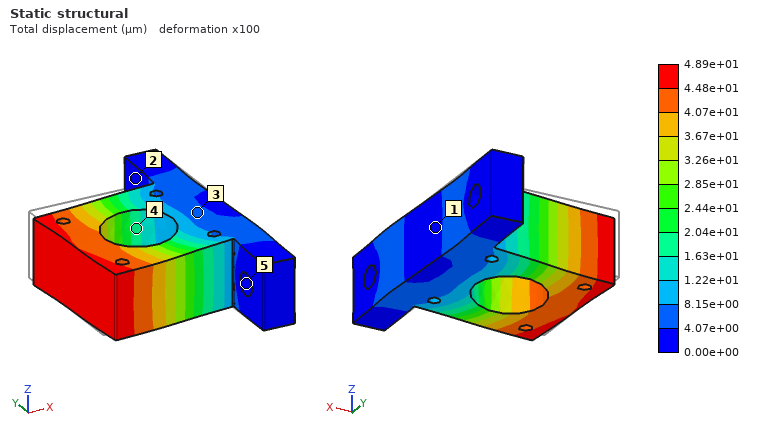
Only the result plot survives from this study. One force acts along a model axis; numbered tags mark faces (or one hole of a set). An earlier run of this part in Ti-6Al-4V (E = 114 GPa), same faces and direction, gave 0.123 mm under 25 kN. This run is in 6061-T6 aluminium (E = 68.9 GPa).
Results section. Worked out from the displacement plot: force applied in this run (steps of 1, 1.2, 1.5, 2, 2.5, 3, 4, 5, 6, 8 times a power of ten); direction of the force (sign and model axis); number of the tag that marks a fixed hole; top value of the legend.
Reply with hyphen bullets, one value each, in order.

- 6 kN
- -Y
- 5
- 4.89e+01 µm
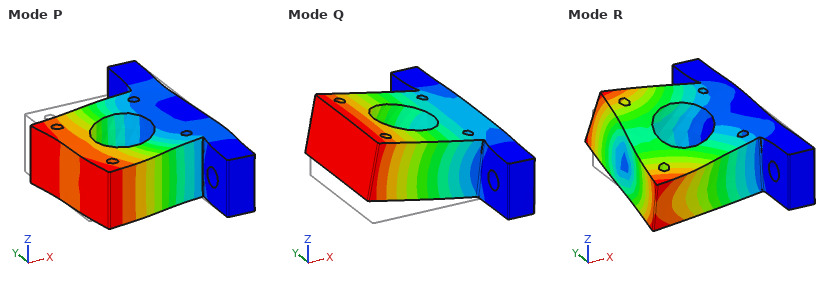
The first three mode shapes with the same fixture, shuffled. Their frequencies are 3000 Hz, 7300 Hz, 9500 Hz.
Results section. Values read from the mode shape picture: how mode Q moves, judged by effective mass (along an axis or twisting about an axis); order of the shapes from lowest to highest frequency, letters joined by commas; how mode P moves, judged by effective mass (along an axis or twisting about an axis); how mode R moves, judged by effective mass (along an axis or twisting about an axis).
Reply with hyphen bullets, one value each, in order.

- along Z
- Q, P, R
- along Y
- twisting about X
